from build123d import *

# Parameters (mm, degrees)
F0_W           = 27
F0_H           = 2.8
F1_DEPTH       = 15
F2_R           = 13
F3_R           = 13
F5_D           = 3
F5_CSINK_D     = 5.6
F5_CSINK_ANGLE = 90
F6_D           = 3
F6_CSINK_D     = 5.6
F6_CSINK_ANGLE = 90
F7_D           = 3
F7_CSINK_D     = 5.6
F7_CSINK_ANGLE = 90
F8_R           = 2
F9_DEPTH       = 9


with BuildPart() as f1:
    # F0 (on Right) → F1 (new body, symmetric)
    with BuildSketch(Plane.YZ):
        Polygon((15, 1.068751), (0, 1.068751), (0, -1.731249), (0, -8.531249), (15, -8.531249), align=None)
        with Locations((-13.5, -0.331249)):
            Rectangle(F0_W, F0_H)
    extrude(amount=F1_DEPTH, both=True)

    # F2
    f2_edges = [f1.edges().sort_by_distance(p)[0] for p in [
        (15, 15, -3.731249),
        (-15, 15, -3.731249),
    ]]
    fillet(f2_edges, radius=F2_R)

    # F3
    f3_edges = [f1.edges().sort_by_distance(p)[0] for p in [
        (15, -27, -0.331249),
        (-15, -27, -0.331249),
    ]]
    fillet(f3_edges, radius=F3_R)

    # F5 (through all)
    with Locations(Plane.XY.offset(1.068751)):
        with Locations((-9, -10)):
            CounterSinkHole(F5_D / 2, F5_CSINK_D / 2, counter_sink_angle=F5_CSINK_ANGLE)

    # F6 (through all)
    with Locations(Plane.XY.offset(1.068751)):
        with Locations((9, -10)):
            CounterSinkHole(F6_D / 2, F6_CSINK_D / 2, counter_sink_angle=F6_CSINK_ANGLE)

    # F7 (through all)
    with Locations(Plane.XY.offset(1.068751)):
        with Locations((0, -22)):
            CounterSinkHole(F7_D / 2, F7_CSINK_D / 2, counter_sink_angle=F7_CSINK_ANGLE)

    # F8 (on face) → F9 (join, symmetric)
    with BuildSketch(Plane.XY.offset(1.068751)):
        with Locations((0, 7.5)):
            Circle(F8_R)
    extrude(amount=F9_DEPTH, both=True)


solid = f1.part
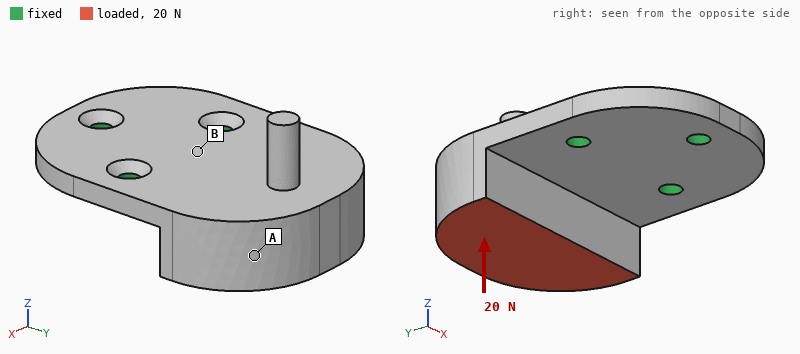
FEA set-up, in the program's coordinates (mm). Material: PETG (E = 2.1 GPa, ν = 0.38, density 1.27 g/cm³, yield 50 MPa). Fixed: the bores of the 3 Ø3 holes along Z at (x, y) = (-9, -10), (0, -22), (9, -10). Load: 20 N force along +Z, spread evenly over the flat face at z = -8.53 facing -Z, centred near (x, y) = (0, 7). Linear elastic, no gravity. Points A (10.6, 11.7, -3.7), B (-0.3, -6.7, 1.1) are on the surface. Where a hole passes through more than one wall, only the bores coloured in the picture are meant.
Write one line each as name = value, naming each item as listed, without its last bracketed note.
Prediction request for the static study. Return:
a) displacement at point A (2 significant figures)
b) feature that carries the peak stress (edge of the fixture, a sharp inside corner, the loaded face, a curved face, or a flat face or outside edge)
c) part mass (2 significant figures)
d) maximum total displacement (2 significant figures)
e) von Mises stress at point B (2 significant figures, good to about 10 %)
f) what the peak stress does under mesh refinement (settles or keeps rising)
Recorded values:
displacement at point A = 0.47 mm
feature that carries the peak stress = edge of the fixture
part mass = 7.3 g
maximum total displacement = 0.58 mm
von Mises stress at point B = 5.7 MPa
what the peak stress does under mesh refinement = keeps rising
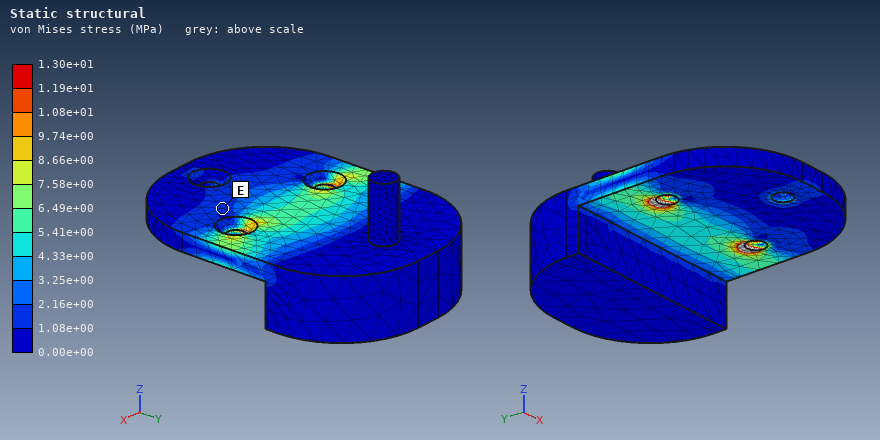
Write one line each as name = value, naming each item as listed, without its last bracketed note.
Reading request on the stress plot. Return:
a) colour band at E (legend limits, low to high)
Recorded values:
colour band at E = 1.08e+00 to 2.16e+00 MPa
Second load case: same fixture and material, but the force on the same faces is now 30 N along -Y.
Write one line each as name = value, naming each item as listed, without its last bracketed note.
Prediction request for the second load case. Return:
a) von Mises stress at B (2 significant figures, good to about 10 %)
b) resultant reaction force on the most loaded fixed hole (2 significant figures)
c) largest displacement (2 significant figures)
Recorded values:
von Mises stress at B = 5.1 MPa
resultant reaction force on the most loaded fixed hole = 20 N
largest displacement = 0.56 mm
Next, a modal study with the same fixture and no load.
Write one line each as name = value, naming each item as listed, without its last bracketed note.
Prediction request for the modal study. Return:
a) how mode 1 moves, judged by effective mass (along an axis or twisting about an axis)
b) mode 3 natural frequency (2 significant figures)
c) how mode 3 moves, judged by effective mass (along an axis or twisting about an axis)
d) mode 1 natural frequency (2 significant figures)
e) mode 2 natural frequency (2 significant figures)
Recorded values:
how mode 1 moves, judged by effective mass = along Z
mode 3 natural frequency = 3300 Hz
how mode 3 moves, judged by effective mass = along X
mode 1 natural frequency = 510 Hz
mode 2 natural frequency = 1800 Hz
